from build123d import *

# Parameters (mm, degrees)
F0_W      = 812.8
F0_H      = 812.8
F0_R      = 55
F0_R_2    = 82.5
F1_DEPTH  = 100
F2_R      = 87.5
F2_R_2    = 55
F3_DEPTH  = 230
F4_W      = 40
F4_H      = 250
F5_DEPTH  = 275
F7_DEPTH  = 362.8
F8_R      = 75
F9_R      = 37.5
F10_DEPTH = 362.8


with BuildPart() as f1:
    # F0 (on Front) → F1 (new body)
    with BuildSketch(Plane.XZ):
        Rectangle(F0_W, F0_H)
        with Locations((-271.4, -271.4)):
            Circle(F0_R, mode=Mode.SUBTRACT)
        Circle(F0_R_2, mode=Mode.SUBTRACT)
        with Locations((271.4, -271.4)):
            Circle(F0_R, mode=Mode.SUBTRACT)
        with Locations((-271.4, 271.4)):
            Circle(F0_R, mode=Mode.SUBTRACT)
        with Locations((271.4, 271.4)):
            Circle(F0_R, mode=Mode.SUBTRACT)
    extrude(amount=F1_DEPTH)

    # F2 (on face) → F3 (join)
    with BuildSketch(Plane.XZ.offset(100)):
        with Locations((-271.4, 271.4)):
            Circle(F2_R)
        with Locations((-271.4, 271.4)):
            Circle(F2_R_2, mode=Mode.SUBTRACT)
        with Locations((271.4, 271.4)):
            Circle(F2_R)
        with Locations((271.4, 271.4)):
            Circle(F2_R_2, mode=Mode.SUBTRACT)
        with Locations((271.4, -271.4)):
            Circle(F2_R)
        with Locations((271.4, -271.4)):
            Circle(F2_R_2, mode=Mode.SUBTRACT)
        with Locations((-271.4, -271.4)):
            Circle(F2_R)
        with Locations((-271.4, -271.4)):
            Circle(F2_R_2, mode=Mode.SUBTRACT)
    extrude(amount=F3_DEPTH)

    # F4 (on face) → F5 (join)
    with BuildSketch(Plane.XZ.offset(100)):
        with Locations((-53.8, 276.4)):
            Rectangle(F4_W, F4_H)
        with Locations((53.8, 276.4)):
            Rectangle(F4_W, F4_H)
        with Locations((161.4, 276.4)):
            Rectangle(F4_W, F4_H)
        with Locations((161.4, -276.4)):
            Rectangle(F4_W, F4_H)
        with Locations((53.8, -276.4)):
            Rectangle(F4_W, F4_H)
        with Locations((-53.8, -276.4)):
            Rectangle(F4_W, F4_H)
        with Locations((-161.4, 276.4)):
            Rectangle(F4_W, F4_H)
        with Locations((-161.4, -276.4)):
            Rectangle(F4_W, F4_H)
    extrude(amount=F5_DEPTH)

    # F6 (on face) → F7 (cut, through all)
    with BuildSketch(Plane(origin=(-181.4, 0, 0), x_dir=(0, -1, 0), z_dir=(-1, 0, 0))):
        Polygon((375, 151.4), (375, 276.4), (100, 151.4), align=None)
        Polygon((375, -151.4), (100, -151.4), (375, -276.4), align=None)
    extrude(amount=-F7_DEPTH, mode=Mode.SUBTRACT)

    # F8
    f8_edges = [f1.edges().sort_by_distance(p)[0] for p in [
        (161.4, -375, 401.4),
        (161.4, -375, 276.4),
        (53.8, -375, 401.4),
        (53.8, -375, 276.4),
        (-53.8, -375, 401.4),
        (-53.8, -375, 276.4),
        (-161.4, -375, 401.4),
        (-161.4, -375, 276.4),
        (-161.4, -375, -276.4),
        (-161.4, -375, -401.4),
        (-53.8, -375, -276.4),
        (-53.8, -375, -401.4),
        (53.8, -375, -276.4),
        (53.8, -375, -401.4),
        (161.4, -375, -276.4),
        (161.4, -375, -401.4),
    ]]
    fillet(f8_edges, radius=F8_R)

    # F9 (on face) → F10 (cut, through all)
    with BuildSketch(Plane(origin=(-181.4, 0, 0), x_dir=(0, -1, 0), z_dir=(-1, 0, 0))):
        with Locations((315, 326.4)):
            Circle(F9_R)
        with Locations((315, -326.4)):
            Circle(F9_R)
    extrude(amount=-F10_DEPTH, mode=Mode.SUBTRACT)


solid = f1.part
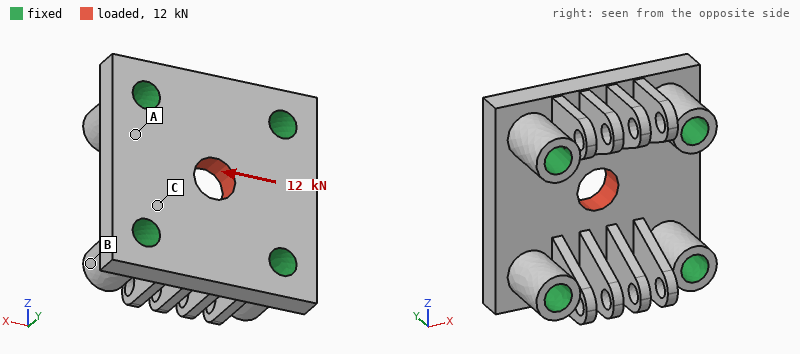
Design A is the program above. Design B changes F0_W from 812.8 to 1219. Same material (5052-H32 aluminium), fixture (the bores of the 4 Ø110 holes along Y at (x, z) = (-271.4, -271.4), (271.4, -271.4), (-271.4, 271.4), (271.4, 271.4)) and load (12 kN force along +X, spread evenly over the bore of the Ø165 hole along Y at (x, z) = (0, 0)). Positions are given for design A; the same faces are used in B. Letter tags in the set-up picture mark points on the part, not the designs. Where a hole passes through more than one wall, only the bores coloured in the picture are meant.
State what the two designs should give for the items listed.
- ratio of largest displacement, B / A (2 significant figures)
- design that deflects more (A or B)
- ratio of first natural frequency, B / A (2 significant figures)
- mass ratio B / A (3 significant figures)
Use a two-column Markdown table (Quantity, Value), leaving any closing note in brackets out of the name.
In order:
| Quantity | Value |
|---|---|
| ratio of largest displacement, B / A | 0.90 |
| design that deflects more | A |
| ratio of first natural frequency, B / A | 1.0 |
| mass ratio B / A | 1.37 |
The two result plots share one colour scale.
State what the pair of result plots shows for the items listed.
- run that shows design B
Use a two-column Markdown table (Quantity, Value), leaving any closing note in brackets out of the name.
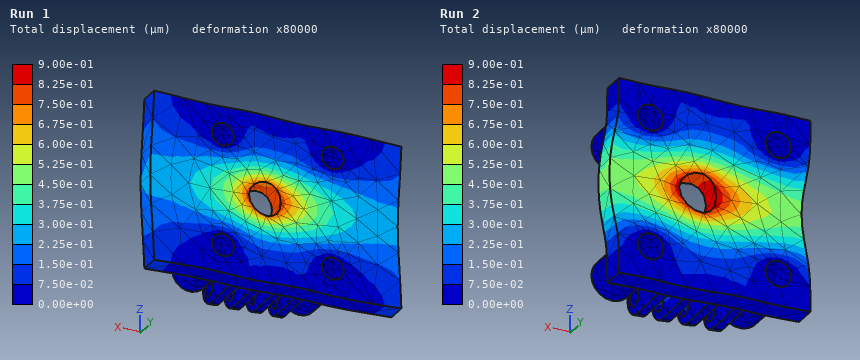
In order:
| Quantity | Value |
|---|---|
| run that shows design B | Run 1 |
